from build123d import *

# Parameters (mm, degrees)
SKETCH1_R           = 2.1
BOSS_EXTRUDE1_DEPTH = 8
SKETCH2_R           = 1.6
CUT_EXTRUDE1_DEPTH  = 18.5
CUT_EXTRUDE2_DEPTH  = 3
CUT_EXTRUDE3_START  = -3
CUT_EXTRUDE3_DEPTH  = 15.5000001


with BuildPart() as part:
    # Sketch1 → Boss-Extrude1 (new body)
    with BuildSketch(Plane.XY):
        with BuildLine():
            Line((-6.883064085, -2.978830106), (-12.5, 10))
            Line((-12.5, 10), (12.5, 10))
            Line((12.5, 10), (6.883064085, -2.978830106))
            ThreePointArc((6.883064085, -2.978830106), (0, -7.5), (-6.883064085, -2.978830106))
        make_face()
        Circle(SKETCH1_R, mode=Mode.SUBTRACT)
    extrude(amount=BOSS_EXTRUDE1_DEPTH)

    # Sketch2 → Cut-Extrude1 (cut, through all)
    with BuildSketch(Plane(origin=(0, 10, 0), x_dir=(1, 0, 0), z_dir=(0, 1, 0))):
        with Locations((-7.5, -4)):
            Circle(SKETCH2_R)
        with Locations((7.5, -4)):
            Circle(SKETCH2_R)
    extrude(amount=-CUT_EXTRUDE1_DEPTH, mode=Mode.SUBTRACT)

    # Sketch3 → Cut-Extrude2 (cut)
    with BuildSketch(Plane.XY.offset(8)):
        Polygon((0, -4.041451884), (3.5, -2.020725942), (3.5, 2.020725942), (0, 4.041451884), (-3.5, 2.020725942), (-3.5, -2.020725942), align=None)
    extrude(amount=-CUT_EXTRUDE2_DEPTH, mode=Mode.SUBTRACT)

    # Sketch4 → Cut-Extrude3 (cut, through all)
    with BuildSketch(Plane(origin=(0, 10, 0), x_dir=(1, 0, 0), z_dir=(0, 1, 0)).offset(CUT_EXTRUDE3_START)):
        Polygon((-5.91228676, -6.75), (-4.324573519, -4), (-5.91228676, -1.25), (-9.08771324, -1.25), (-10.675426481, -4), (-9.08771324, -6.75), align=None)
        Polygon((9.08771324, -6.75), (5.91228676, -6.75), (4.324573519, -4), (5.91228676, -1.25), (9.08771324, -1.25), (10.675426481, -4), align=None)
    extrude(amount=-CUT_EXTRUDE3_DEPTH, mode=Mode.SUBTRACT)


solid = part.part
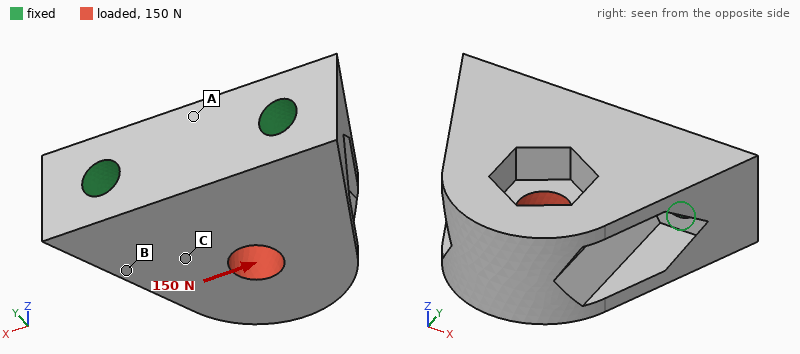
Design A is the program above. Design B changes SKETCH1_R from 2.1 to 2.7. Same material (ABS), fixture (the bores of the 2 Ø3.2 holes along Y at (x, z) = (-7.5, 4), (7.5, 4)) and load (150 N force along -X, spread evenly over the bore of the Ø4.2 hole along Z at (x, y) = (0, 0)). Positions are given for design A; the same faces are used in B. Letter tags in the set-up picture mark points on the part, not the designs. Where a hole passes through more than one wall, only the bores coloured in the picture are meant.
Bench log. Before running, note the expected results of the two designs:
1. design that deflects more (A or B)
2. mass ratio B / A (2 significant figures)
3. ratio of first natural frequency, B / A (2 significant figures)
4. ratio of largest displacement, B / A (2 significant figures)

B
0.97
1.0
1.1
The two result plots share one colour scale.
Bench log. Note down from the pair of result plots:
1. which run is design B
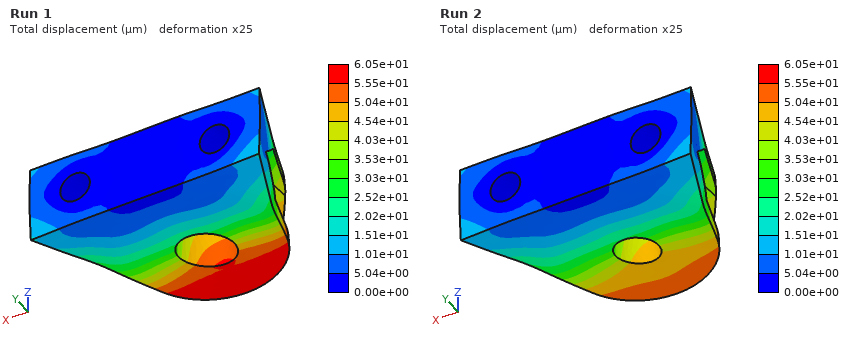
Run 1
